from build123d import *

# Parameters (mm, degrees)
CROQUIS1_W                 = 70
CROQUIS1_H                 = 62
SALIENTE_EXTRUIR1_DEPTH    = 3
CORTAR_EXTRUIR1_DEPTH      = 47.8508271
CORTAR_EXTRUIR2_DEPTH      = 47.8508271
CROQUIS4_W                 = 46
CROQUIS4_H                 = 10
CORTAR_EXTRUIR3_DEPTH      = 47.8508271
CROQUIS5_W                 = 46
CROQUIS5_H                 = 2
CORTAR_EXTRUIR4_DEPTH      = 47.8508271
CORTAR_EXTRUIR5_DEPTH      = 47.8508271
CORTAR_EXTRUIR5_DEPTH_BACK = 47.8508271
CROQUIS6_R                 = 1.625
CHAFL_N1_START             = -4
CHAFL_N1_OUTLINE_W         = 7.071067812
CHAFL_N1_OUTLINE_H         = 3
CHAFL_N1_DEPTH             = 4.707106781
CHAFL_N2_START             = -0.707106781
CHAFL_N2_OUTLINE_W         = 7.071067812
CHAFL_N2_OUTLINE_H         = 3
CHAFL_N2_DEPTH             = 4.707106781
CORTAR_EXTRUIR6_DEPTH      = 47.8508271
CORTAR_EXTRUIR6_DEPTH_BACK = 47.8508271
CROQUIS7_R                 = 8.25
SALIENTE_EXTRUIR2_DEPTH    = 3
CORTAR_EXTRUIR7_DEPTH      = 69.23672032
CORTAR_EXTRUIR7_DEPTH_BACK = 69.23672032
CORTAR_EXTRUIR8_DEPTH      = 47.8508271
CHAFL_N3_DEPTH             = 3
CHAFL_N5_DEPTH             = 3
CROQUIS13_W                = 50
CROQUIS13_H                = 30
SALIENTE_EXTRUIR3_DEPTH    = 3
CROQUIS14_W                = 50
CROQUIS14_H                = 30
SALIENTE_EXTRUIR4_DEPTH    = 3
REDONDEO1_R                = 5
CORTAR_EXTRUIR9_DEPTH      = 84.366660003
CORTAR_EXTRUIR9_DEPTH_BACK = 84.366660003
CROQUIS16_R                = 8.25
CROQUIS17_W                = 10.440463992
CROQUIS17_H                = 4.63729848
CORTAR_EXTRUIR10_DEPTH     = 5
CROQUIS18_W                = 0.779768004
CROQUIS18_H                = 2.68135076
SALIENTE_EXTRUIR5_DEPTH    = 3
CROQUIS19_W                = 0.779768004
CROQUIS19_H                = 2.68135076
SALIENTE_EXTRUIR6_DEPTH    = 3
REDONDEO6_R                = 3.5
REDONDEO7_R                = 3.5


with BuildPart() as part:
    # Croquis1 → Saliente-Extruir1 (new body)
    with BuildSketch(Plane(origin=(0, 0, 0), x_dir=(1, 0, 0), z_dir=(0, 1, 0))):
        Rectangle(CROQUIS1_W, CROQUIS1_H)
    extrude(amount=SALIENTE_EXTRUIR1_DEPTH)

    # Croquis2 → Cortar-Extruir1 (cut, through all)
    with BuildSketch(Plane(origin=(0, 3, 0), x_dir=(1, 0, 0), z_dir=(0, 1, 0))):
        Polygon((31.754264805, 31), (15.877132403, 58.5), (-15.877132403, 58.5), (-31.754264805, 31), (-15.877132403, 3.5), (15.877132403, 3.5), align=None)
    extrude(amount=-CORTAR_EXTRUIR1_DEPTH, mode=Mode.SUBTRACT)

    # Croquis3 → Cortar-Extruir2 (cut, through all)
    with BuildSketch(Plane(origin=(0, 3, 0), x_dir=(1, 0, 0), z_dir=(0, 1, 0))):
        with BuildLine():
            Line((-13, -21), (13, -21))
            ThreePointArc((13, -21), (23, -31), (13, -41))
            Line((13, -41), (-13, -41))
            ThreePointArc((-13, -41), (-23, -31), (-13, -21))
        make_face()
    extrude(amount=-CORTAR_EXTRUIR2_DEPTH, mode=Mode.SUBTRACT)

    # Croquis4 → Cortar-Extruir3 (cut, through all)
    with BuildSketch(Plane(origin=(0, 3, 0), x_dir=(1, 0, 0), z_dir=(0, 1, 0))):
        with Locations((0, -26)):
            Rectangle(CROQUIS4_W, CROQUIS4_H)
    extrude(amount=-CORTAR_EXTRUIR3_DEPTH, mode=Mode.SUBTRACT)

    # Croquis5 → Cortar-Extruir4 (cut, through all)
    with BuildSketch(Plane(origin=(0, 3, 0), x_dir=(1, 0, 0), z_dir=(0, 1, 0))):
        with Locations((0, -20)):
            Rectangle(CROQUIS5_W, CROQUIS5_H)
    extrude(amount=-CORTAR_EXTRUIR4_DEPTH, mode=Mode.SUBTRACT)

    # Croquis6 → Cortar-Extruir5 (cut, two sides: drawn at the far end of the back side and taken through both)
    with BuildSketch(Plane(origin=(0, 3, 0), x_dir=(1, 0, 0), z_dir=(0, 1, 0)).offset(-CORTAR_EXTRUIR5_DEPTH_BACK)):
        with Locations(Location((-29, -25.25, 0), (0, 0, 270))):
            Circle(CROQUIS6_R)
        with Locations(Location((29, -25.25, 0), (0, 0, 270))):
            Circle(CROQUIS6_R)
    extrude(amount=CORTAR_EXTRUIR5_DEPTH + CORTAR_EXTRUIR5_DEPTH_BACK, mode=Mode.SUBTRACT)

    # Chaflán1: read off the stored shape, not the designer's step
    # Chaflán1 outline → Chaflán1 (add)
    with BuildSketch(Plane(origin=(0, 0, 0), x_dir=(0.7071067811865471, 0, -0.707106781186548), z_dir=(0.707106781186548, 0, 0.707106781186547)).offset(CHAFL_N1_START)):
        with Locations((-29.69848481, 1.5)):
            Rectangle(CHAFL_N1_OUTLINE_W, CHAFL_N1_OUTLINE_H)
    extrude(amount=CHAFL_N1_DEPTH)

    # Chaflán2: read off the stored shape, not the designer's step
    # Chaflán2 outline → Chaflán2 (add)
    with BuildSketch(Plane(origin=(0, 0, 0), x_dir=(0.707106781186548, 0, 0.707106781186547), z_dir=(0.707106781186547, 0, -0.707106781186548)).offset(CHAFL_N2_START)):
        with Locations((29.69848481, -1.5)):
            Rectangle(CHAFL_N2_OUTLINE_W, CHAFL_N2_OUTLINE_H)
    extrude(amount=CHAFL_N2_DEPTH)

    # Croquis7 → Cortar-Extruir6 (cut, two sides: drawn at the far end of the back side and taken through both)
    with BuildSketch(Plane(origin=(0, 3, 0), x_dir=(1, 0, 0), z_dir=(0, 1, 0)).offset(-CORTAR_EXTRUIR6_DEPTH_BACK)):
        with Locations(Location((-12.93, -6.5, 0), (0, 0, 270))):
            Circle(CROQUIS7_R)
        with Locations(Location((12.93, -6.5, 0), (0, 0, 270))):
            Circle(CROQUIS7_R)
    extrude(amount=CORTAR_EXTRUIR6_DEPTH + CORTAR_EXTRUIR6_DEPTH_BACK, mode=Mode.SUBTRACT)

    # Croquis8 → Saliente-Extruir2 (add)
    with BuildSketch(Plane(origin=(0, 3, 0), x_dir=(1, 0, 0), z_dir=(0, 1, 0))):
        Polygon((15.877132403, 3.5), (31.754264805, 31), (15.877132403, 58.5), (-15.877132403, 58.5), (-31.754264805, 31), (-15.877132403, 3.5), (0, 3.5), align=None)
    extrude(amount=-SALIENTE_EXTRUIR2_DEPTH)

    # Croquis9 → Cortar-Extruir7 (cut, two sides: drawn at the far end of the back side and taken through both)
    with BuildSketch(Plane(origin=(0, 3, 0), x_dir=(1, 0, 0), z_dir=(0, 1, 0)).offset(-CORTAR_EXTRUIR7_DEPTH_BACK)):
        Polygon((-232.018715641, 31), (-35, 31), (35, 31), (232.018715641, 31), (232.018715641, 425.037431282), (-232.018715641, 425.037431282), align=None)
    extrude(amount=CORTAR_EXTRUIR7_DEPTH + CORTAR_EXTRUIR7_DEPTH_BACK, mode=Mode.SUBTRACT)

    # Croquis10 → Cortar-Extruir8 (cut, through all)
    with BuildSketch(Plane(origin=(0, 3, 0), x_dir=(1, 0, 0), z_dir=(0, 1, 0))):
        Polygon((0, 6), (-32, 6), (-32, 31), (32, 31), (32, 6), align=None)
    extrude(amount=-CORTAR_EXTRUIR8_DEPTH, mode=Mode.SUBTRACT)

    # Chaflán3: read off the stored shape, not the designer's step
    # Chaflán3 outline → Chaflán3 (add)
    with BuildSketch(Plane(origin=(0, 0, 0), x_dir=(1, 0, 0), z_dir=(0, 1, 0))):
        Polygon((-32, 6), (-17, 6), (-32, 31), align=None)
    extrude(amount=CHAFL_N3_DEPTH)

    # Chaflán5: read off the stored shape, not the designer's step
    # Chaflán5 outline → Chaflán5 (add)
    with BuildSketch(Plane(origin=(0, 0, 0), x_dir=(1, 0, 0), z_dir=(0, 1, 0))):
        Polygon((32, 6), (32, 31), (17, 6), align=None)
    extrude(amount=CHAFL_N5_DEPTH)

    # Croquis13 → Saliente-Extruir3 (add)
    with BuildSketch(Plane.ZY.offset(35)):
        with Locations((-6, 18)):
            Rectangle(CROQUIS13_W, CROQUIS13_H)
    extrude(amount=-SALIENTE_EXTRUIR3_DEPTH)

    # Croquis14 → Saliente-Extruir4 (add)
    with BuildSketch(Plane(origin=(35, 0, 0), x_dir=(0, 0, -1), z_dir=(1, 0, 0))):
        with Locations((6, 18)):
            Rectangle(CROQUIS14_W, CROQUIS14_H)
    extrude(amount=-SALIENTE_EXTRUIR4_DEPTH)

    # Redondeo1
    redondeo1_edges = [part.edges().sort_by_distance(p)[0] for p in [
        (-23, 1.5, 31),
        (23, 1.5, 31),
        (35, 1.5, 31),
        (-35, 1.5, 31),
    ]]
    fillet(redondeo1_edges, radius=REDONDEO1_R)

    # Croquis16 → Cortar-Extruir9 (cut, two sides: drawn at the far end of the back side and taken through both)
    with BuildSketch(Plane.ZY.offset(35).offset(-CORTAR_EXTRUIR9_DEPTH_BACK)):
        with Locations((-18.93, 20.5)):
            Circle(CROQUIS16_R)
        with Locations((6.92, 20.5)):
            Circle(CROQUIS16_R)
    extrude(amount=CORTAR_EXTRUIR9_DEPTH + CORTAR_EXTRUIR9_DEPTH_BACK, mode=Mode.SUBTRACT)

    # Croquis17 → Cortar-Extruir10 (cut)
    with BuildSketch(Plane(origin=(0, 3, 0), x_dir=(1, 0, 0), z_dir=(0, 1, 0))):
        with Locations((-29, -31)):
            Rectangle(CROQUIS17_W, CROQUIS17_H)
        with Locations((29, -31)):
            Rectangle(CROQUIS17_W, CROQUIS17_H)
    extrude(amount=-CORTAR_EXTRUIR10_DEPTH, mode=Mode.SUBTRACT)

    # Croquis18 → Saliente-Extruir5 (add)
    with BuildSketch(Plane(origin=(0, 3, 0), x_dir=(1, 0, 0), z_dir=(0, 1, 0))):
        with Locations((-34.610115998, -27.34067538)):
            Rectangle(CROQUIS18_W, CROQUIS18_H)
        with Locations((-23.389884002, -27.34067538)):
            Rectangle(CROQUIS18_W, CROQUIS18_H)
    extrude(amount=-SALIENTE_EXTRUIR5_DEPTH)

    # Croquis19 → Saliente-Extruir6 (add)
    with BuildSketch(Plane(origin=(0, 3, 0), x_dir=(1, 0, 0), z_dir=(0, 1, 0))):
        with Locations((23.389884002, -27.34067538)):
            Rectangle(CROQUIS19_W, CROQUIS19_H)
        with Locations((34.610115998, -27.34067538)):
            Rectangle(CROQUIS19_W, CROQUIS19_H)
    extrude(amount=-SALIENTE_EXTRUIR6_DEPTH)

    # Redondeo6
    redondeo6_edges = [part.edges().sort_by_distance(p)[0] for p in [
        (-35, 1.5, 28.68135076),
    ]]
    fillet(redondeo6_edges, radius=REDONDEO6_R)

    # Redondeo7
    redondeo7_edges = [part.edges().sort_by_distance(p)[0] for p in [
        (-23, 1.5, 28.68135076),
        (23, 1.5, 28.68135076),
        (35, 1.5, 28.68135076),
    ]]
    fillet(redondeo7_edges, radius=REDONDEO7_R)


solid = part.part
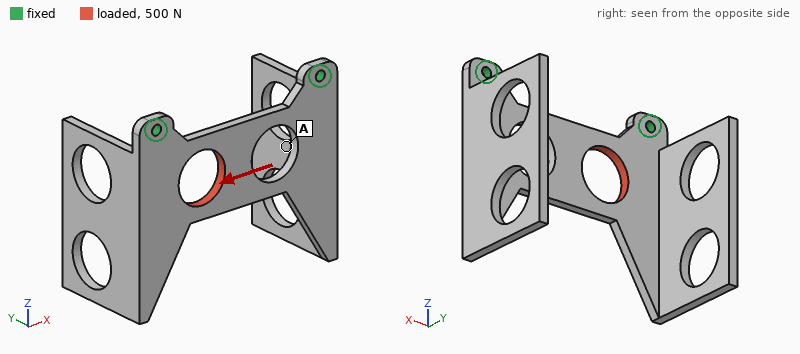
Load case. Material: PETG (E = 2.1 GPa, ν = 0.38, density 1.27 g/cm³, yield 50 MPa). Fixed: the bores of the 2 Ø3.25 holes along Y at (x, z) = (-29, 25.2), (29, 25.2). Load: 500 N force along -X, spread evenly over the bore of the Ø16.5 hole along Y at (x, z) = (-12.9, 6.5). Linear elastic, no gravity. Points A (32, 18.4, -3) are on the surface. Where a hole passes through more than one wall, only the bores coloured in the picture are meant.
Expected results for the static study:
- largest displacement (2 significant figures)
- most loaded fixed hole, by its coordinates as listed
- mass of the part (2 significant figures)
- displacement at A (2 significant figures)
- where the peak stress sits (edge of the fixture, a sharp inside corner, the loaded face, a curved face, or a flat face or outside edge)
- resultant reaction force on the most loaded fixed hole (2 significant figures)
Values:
0.83 mm
(-29, 25.2)
16 g
0.38 mm
edge of the fixture
300 N
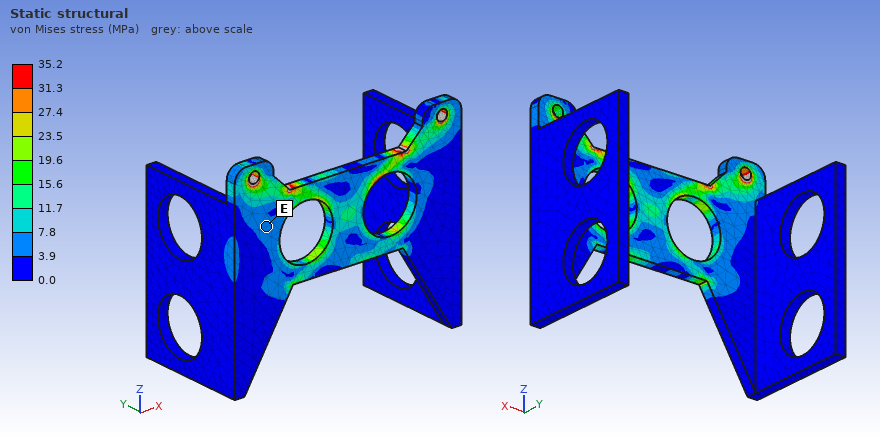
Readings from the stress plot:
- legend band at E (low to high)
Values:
3.9 to 7.8 MPa
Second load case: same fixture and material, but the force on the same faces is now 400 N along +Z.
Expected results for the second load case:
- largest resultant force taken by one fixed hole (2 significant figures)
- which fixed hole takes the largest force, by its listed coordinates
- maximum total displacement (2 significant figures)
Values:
310 N
(-29, 25.2)
0.37 mm
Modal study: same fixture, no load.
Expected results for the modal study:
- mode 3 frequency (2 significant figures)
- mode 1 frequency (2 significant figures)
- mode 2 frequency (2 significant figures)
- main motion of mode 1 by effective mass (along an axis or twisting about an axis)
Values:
300 Hz
150 Hz
180 Hz
along Y
